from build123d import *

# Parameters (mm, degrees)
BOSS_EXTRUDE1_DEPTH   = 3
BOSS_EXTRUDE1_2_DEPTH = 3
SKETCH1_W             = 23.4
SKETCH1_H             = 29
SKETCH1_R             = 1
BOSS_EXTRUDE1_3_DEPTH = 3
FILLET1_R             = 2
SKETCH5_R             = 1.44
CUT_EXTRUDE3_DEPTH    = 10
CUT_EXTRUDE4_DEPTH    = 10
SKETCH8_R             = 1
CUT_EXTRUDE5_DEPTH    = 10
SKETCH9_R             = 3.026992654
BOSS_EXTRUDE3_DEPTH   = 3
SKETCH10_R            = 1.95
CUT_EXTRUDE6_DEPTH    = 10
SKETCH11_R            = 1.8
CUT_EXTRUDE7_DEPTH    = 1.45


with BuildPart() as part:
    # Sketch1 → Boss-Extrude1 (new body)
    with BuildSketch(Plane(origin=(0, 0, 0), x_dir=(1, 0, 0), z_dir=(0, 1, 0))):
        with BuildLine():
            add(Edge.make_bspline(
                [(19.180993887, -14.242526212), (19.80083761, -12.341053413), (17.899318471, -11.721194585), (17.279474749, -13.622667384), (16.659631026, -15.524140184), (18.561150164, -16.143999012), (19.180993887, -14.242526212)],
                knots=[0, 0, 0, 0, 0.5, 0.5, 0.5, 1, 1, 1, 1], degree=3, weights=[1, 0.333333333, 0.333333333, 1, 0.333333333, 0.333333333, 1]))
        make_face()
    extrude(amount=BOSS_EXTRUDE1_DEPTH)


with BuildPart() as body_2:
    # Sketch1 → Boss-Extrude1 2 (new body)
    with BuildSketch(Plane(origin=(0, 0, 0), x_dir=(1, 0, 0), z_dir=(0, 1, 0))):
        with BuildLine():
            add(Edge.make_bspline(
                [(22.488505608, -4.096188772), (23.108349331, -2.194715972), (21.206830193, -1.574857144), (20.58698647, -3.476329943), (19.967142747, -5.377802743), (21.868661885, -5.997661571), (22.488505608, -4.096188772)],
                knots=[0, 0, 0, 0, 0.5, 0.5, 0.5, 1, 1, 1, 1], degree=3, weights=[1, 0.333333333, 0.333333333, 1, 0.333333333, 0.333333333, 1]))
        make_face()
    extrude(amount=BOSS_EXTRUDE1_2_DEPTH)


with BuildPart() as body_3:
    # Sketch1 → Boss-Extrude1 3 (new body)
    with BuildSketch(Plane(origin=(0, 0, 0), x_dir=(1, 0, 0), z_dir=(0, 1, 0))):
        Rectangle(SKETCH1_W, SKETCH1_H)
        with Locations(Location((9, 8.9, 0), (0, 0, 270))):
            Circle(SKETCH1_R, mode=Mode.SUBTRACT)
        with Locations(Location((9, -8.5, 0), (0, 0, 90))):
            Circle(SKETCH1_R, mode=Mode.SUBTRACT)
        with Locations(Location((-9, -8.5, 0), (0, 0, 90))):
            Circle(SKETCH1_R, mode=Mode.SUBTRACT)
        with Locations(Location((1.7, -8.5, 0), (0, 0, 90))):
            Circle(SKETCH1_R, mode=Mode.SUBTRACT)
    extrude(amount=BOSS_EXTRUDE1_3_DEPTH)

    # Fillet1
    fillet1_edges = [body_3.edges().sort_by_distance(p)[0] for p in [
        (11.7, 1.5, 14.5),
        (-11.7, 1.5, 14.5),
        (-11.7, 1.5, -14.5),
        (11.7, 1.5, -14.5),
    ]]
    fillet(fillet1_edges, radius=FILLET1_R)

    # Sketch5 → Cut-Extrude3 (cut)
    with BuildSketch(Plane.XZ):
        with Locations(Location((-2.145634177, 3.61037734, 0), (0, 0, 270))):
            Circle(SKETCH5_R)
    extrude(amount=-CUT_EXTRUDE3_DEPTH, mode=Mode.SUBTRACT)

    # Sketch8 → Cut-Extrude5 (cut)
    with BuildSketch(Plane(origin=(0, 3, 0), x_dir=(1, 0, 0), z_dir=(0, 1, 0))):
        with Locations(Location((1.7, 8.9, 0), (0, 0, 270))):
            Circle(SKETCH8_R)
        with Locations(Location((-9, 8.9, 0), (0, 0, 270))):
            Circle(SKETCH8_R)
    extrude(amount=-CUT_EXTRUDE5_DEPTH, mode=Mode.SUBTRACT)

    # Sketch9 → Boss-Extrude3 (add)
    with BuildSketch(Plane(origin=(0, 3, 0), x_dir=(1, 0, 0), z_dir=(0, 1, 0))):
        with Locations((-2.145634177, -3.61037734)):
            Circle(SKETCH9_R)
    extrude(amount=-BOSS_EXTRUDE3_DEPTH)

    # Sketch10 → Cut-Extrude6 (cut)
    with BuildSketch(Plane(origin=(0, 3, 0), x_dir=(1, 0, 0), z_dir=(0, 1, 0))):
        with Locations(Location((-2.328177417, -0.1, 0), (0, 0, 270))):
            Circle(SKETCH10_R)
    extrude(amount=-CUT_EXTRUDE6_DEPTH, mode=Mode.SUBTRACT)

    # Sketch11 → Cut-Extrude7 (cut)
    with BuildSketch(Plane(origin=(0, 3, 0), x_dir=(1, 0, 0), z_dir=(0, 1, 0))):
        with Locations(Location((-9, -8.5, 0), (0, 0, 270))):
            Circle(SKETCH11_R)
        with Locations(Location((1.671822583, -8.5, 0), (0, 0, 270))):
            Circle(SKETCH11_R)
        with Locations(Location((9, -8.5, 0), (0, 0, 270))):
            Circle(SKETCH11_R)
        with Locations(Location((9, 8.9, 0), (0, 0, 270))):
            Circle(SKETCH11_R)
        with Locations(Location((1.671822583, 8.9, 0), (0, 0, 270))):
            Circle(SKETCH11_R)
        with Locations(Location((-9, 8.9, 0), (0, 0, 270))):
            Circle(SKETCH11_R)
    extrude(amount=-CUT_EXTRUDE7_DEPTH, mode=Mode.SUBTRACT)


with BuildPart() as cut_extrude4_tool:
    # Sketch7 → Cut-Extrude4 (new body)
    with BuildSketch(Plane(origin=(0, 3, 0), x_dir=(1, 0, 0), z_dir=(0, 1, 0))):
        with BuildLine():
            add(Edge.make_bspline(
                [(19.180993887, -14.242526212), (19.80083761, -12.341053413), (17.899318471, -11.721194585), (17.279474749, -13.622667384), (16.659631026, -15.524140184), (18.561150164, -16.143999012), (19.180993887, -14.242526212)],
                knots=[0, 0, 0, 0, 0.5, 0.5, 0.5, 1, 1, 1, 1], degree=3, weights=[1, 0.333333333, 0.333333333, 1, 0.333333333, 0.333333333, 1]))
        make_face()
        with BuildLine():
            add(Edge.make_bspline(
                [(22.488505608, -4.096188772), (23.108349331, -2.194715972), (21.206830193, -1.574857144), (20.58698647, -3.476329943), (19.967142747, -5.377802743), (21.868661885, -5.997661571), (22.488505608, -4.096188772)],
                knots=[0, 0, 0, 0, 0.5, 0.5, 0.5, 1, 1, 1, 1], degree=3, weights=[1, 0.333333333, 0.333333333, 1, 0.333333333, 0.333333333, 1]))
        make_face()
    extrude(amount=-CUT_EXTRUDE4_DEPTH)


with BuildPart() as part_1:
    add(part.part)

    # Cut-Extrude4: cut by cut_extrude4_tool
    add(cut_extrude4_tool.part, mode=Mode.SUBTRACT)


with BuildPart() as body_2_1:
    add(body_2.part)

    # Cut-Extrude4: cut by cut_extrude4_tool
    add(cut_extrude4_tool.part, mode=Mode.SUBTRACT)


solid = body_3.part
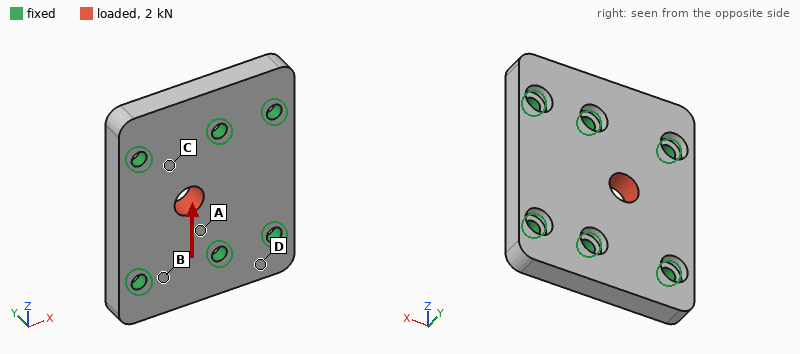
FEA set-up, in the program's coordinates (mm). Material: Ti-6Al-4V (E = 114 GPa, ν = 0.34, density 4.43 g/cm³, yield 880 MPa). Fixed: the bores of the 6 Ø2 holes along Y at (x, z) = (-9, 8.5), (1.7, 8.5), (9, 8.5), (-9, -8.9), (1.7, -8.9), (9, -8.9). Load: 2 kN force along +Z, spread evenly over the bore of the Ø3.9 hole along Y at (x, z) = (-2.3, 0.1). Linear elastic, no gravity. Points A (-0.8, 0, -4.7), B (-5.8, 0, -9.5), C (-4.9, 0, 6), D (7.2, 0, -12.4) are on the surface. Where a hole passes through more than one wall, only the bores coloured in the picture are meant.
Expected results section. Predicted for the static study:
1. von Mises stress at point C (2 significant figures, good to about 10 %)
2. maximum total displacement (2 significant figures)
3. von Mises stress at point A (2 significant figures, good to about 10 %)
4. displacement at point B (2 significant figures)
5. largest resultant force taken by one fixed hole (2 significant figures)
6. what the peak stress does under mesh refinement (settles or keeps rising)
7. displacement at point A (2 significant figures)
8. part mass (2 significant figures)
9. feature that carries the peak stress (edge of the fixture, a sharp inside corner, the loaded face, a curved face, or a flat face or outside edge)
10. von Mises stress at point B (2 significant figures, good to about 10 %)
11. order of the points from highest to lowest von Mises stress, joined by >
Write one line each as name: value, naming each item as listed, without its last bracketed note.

von Mises stress at point C: 31 MPa
maximum total displacement: 3.5 µm
von Mises stress at point A: 45 MPa
displacement at point B: 0.91 µm
largest resultant force taken by one fixed hole: 500 N
what the peak stress does under mesh refinement: keeps rising
displacement at point A: 1.9 µm
part mass: 8.3 g
feature that carries the peak stress: edge of the fixture
von Mises stress at point B: 16 MPa
order of the points from highest to lowest von Mises stress, joined by >: A > C > B > D
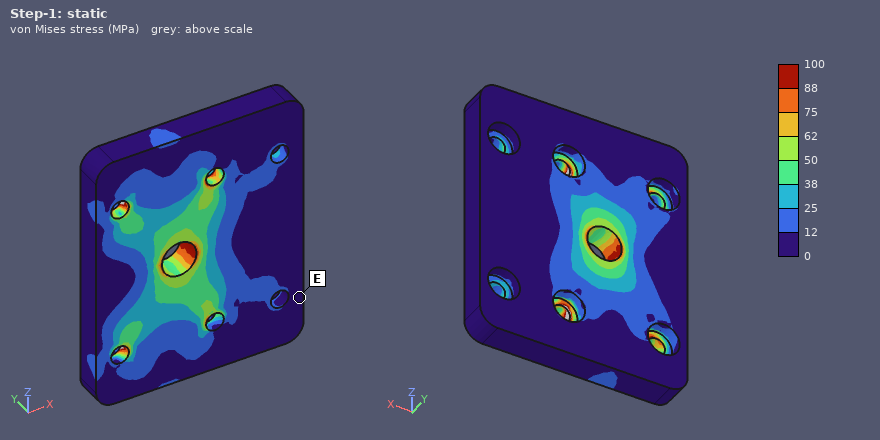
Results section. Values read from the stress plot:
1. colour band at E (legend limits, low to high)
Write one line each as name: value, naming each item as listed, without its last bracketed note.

colour band at E: 0 to 12 MPa
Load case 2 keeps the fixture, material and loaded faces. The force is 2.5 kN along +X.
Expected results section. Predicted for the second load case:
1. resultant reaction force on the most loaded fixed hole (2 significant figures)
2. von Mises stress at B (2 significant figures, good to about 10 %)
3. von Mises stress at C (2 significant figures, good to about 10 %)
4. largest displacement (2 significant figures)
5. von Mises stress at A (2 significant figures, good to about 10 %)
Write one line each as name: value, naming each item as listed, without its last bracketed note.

resultant reaction force on the most loaded fixed hole: 540 N
von Mises stress at B: 17 MPa
von Mises stress at C: 43 MPa
largest displacement: 6.1 µm
von Mises stress at A: 44 MPa
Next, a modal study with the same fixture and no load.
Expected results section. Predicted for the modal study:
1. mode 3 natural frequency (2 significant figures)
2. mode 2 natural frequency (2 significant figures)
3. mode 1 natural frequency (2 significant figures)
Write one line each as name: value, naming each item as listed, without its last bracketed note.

mode 3 natural frequency: 41 kHz
mode 2 natural frequency: 40 kHz
mode 1 natural frequency: 32 kHz
